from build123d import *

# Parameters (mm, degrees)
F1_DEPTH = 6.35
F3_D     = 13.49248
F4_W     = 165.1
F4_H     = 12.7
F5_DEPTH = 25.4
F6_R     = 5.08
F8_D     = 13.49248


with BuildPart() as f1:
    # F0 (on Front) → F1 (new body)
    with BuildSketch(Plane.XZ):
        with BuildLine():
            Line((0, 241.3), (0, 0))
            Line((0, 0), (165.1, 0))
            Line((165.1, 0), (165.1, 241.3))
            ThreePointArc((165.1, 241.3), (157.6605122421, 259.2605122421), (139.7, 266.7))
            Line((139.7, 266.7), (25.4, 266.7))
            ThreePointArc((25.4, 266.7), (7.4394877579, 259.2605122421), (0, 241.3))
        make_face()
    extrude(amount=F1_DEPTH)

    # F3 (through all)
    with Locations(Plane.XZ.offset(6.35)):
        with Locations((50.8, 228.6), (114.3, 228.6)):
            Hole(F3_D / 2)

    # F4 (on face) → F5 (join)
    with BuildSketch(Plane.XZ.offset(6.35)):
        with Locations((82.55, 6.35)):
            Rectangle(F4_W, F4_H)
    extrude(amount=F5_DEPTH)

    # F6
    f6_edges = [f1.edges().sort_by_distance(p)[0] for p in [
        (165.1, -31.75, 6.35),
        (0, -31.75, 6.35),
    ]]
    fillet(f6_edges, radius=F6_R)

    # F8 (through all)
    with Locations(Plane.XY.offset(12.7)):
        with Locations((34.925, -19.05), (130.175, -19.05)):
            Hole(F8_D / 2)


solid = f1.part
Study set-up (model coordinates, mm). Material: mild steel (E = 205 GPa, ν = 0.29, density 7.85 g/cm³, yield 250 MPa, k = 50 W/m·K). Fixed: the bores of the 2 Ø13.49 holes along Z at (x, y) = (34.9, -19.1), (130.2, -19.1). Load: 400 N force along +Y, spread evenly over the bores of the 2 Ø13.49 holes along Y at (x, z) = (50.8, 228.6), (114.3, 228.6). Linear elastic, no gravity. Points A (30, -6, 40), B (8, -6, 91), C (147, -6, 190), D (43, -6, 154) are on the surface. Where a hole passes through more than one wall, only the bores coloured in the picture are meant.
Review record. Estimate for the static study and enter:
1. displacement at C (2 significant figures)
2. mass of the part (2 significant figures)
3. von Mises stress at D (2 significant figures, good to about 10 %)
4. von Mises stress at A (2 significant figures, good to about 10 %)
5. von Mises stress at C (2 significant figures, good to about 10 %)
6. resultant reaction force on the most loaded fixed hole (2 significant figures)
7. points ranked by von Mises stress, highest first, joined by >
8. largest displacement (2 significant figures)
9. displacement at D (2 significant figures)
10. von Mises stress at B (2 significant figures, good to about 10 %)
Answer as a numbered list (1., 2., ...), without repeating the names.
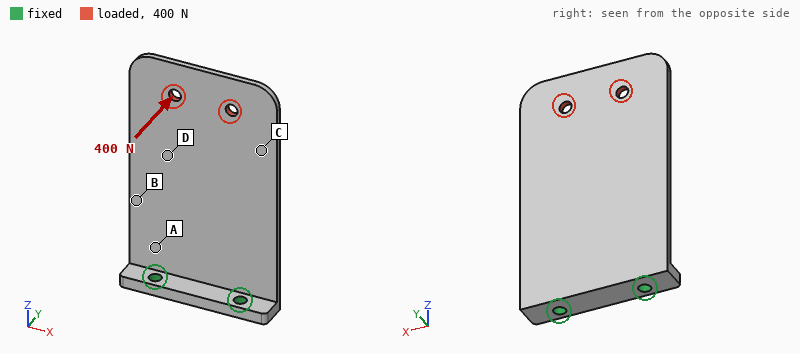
1. 1.4 mm
2. 2.6 kg
3. 27 MPa
4. 61 MPa
5. 14 MPa
6. 230 N
7. A > B > D > C
8. 2.4 mm
9. 0.98 mm
10. 50 MPa
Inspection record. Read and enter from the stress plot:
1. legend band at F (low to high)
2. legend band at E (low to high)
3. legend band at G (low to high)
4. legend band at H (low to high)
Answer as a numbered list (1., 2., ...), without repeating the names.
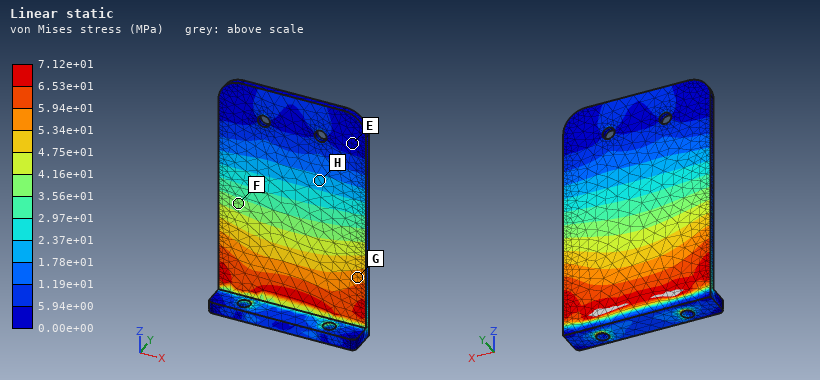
1. 3.56e+01 to 4.16e+01 MPa
2. 0.00e+00 to 5.94e+00 MPa
3. 5.34e+01 to 5.94e+01 MPa
4. 1.78e+01 to 2.37e+01 MPa
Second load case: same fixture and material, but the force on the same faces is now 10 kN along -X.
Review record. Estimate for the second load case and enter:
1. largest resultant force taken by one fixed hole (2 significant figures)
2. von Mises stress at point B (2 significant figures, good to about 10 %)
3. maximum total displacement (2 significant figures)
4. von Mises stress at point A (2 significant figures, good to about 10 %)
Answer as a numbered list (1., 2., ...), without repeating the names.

1. 22 kN
2. 47 MPa
3. 0.27 mm
4. 66 MPa
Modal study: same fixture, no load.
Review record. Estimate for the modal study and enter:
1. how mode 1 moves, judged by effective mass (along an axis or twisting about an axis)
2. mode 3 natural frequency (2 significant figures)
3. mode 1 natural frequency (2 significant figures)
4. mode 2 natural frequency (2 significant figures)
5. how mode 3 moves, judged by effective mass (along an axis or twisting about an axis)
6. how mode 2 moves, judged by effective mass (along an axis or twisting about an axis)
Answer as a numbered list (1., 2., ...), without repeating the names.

1. along Y
2. 500 Hz
3. 81 Hz
4. 280 Hz
5. along Y
6. twisting about Z
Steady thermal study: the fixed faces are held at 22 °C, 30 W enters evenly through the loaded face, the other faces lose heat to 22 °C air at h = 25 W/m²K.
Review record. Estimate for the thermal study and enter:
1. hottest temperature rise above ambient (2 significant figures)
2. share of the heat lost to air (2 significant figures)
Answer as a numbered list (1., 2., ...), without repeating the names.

1. 39 K
2. 93 %
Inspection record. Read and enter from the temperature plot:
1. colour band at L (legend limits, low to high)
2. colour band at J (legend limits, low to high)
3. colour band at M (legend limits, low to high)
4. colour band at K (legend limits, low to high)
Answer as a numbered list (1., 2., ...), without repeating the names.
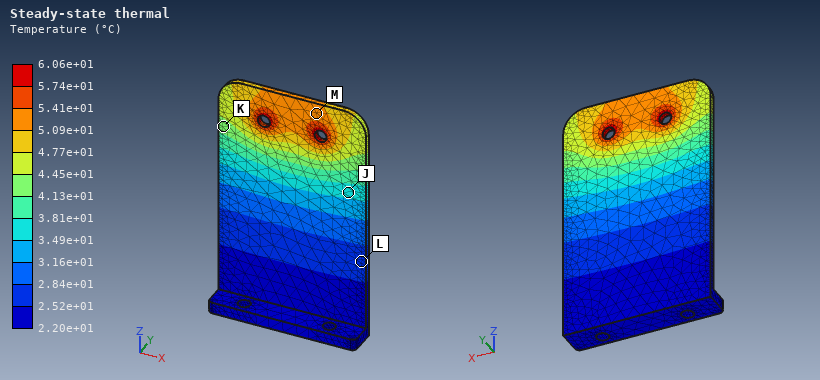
1. 2.52e+01 to 2.84e+01 °C
2. 3.49e+01 to 3.81e+01 °C
3. 5.09e+01 to 5.41e+01 °C
4. 4.13e+01 to 4.45e+01 °C
